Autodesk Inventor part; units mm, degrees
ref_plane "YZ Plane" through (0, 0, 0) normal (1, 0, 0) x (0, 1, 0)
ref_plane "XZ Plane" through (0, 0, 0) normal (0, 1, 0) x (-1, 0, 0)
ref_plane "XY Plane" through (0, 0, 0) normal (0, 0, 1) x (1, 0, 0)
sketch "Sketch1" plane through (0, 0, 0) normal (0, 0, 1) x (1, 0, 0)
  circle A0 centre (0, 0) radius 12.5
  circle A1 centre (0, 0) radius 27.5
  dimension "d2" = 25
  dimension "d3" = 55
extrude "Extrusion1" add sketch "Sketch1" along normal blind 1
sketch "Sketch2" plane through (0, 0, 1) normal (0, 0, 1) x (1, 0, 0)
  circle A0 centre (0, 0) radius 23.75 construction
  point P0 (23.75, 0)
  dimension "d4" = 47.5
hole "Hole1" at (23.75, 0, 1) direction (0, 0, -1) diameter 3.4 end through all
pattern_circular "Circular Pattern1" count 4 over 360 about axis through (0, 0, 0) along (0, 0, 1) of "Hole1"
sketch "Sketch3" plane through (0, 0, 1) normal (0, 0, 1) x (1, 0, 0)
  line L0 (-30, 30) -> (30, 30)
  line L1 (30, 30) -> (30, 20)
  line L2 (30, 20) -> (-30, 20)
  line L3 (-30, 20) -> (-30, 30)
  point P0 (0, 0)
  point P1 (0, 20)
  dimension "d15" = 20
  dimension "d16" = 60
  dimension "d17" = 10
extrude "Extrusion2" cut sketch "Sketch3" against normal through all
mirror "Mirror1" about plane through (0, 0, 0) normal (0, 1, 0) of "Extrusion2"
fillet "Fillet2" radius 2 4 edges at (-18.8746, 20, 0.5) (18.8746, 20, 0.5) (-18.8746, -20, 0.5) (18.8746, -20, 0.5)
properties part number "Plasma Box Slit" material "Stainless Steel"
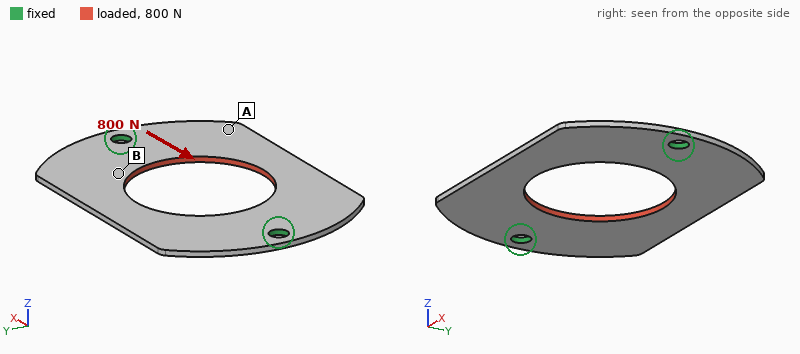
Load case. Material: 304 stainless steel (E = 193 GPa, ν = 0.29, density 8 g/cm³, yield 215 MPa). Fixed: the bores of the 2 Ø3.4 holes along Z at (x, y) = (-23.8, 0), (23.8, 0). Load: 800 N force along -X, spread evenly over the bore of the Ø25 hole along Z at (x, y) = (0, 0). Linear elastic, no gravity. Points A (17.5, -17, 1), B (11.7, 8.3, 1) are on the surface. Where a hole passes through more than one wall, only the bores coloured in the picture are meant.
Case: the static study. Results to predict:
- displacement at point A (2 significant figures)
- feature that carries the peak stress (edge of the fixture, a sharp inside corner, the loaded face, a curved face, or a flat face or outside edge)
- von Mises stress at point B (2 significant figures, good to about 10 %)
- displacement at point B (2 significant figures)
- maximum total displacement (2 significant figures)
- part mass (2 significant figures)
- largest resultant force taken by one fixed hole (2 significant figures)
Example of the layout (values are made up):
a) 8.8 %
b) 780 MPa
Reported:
a) 3.4 µm
b) edge of the fixture
c) 22 MPa
d) 2.9 µm
e) 4.2 µm
f) 12 g
g) 400 N
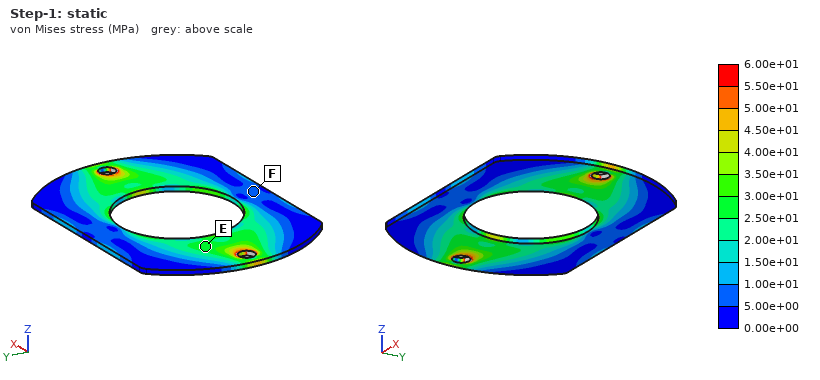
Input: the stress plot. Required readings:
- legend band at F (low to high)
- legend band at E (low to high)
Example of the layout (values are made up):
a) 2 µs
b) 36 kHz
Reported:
a) 5.00e+00 to 1.00e+01 MPa
b) 2.50e+01 to 3.00e+01 MPa
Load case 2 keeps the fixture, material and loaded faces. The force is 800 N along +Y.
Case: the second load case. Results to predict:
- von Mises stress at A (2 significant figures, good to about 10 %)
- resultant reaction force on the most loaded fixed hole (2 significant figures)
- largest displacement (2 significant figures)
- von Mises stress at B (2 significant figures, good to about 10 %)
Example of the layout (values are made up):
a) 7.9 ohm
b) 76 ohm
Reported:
a) 8.2 MPa
b) 400 N
c) 5.7 µm
d) 25 MPa
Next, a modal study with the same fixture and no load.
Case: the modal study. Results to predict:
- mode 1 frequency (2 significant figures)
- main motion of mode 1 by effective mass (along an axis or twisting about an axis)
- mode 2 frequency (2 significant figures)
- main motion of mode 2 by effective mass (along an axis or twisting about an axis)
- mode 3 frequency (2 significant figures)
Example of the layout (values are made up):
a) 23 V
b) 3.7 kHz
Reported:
a) 1300 Hz
b) twisting about X
c) 1500 Hz
d) along Z
e) 2800 Hz
